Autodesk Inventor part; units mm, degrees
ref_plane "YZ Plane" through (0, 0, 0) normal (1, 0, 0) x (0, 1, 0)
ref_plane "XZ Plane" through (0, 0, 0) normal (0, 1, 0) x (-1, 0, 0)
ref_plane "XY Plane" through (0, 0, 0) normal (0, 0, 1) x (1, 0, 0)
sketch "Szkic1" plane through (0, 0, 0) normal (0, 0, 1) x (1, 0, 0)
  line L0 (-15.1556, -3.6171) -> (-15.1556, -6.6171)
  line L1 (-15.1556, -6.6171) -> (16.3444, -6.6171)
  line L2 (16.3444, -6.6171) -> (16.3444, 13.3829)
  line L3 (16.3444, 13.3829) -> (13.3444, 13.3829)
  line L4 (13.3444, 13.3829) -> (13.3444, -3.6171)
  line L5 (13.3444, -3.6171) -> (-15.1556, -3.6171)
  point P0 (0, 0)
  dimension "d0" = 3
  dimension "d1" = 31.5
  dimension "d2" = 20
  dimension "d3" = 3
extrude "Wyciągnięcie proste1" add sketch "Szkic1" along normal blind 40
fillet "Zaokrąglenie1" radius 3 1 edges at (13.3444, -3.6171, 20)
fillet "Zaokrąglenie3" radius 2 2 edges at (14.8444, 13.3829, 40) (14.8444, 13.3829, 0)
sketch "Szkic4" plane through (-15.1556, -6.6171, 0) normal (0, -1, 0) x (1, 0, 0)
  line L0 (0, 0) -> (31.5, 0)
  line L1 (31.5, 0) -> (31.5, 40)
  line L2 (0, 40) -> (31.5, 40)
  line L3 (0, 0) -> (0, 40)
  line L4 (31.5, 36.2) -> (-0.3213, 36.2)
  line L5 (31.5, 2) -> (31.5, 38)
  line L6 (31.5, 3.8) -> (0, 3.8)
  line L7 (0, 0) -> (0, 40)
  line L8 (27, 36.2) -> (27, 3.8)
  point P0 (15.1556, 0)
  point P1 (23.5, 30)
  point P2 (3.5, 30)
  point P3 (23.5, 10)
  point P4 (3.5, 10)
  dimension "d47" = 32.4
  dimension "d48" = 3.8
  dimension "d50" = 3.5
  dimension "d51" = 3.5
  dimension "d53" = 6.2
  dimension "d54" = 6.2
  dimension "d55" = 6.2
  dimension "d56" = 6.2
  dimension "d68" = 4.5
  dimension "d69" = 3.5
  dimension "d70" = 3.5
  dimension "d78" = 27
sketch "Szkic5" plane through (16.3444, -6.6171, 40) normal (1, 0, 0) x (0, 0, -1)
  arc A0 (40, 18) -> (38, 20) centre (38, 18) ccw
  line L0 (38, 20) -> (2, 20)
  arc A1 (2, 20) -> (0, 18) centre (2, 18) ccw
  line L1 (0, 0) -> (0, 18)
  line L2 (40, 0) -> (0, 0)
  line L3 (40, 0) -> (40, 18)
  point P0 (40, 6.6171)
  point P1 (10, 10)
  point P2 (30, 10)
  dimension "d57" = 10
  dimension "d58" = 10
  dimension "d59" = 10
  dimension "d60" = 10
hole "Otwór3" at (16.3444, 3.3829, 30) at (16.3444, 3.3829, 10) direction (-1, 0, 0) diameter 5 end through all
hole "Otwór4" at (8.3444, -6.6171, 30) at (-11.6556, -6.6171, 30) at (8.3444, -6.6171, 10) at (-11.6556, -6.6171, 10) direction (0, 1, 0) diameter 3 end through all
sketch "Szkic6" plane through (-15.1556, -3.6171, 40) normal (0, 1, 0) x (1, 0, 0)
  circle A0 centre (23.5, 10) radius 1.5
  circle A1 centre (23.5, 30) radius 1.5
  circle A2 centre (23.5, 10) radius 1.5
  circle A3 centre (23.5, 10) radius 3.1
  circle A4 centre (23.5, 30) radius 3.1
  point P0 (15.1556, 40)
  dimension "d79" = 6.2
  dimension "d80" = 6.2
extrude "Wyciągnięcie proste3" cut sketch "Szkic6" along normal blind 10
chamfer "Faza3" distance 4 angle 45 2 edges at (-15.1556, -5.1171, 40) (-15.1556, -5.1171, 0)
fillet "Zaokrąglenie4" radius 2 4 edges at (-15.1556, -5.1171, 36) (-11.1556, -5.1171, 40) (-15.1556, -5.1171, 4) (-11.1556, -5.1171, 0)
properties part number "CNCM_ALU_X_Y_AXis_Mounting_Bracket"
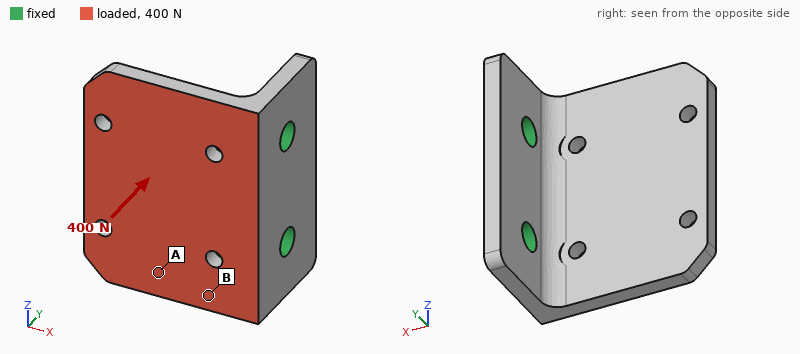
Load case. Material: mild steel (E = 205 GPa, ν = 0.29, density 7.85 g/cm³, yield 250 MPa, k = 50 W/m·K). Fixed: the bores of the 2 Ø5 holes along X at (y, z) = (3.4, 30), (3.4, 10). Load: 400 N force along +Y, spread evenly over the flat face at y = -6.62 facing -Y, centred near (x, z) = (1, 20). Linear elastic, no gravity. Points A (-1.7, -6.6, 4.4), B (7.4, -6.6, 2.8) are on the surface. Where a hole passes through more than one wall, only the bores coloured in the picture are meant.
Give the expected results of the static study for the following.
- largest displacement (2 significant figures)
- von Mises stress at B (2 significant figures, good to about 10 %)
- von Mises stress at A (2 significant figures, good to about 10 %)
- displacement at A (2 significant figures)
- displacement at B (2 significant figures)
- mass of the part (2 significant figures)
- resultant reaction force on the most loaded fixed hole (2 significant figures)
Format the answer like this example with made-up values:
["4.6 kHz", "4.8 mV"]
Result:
["0.10 mm", "55 MPa", "18 MPa", "0.050 mm", "0.020 mm", "44 g", "200 N"]
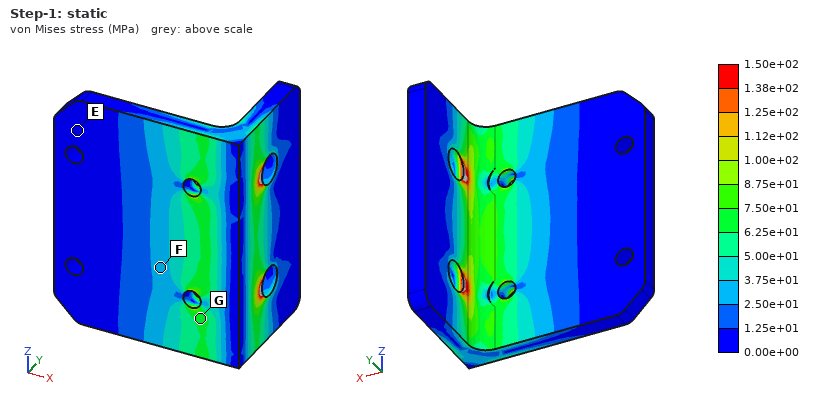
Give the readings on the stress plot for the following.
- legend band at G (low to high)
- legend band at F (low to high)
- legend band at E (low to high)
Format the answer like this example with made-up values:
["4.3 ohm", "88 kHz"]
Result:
["6.25e+01 to 7.50e+01 MPa", "2.50e+01 to 3.75e+01 MPa", "0.00e+00 to 1.25e+01 MPa"]
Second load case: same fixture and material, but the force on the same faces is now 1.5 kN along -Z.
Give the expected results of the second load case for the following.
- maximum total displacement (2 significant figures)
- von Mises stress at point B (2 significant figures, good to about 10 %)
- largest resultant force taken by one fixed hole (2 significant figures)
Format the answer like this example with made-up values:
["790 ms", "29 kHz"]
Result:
["32 µm", "26 MPa", "1.3 kN"]
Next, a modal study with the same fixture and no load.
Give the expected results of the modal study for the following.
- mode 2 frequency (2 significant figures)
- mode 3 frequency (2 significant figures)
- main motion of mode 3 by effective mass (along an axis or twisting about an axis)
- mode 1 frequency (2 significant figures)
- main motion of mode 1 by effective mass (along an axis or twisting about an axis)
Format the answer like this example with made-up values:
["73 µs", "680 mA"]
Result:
["4900 Hz", "7800 Hz", "along Z", "2300 Hz", "along Y"]
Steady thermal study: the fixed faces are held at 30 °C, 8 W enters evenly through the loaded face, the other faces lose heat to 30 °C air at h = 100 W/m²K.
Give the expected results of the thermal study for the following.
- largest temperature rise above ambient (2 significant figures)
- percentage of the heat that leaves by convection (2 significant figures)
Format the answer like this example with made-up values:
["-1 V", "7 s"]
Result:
["18 K", "32 %"]
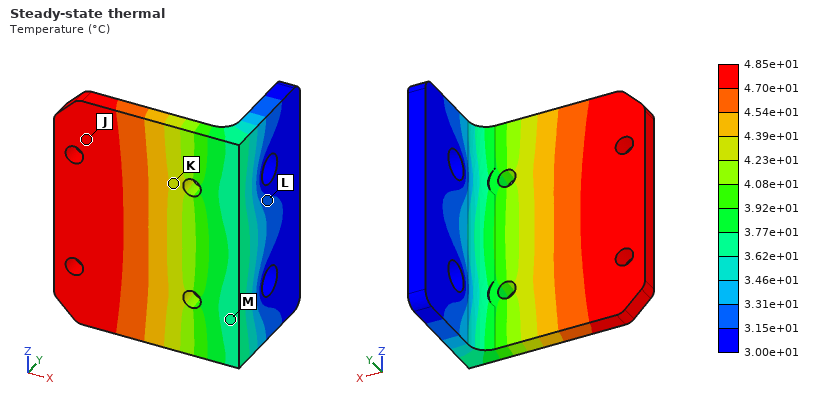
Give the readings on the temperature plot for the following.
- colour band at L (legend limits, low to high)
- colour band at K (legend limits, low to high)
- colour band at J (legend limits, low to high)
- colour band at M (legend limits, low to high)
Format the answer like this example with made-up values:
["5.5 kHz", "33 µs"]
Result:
["3.15e+01 to 3.31e+01 °C", "4.23e+01 to 4.39e+01 °C", "4.70e+01 to 4.85e+01 °C", "3.62e+01 to 3.77e+01 °C"]
